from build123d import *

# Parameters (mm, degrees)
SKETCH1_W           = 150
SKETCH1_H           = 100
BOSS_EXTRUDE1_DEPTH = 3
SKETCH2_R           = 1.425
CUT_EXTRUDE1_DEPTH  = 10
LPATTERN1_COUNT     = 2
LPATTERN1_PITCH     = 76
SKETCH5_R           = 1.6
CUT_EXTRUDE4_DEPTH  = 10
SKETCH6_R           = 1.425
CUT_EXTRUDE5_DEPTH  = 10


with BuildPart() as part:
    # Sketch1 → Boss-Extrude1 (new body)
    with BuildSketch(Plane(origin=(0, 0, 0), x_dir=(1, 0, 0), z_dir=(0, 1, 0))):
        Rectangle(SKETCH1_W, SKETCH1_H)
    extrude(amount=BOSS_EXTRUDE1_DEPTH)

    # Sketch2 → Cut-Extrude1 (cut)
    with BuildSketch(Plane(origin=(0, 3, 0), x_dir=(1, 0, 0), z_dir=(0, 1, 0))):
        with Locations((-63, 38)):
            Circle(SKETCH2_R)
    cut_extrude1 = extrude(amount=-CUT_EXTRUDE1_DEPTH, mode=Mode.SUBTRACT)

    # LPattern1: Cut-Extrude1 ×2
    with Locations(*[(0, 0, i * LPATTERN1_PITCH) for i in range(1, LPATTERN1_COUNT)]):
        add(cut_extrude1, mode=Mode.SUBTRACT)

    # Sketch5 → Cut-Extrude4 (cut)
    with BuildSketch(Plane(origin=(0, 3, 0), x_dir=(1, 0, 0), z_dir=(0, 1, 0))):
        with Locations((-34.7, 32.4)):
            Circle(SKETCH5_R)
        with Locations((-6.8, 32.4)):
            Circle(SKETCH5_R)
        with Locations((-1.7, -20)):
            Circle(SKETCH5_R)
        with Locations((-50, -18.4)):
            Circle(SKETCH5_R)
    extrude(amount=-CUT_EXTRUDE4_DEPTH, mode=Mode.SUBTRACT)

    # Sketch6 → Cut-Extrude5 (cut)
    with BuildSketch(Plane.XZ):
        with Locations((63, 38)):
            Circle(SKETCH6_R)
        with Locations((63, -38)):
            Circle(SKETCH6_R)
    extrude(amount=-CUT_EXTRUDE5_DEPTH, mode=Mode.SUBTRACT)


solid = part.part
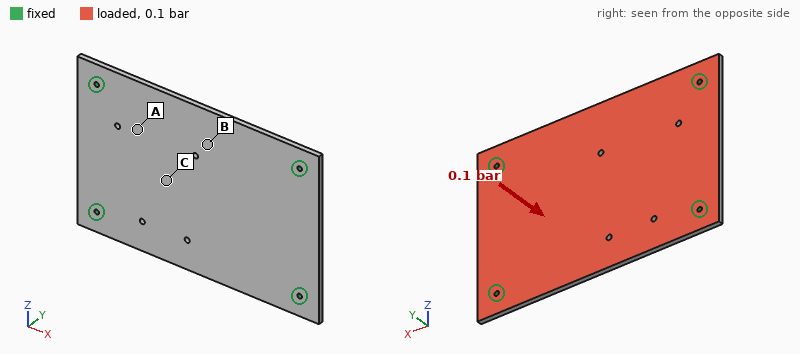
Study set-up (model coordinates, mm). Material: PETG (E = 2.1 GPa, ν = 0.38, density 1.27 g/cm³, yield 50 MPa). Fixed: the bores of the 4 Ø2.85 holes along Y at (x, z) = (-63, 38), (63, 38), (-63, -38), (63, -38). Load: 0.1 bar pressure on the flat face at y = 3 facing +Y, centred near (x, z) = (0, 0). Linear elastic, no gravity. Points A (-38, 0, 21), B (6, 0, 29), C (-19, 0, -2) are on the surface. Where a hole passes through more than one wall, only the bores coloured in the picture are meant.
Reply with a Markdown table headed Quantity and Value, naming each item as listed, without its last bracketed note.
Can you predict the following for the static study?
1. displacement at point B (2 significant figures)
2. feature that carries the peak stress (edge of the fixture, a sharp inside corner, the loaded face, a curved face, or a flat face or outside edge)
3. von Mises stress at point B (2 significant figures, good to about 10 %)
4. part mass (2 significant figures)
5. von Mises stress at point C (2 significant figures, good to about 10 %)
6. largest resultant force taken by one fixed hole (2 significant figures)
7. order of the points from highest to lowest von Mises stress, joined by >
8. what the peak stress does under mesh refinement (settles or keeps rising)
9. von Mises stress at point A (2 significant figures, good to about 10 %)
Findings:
| Quantity | Value |
|---|---|
| displacement at point B | 1.9 mm |
| feature that carries the peak stress | edge of the fixture |
| von Mises stress at point B | 4.9 MPa |
| part mass | 57 g |
| von Mises stress at point C | 3.8 MPa |
| largest resultant force taken by one fixed hole | 37 N |
| order of the points from highest to lowest von Mises stress, joined by > | B > C > A |
| what the peak stress does under mesh refinement | keeps rising |
| von Mises stress at point A | 1.6 MPa |
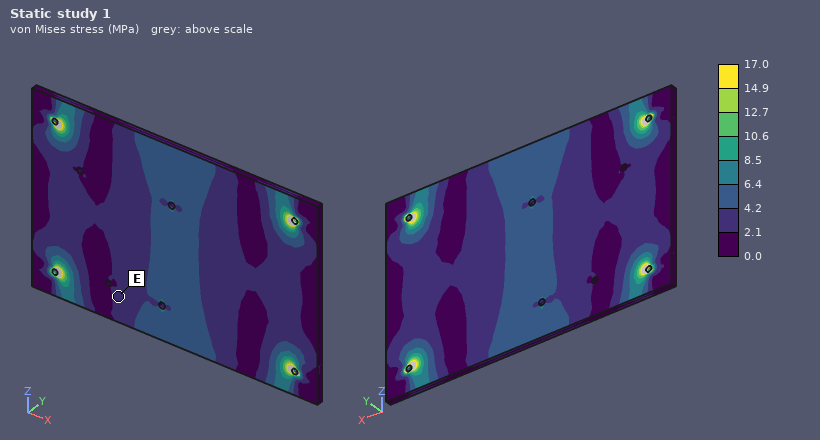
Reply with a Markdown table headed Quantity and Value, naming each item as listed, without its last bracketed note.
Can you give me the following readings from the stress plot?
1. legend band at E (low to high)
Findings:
| Quantity | Value |
|---|---|
| legend band at E | 2.1 to 4.2 MPa |
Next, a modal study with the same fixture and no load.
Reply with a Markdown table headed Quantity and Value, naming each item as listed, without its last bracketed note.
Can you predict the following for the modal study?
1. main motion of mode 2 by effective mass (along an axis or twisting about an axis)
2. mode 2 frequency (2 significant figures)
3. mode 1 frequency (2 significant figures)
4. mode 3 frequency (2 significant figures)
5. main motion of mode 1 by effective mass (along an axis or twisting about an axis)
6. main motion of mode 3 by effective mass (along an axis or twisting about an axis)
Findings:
| Quantity | Value |
|---|---|
| main motion of mode 2 by effective mass | twisting about X |
| mode 2 frequency | 310 Hz |
| mode 1 frequency | 210 Hz |
| mode 3 frequency | 540 Hz |
| main motion of mode 1 by effective mass | along Y |
| main motion of mode 3 by effective mass | twisting about Z |
